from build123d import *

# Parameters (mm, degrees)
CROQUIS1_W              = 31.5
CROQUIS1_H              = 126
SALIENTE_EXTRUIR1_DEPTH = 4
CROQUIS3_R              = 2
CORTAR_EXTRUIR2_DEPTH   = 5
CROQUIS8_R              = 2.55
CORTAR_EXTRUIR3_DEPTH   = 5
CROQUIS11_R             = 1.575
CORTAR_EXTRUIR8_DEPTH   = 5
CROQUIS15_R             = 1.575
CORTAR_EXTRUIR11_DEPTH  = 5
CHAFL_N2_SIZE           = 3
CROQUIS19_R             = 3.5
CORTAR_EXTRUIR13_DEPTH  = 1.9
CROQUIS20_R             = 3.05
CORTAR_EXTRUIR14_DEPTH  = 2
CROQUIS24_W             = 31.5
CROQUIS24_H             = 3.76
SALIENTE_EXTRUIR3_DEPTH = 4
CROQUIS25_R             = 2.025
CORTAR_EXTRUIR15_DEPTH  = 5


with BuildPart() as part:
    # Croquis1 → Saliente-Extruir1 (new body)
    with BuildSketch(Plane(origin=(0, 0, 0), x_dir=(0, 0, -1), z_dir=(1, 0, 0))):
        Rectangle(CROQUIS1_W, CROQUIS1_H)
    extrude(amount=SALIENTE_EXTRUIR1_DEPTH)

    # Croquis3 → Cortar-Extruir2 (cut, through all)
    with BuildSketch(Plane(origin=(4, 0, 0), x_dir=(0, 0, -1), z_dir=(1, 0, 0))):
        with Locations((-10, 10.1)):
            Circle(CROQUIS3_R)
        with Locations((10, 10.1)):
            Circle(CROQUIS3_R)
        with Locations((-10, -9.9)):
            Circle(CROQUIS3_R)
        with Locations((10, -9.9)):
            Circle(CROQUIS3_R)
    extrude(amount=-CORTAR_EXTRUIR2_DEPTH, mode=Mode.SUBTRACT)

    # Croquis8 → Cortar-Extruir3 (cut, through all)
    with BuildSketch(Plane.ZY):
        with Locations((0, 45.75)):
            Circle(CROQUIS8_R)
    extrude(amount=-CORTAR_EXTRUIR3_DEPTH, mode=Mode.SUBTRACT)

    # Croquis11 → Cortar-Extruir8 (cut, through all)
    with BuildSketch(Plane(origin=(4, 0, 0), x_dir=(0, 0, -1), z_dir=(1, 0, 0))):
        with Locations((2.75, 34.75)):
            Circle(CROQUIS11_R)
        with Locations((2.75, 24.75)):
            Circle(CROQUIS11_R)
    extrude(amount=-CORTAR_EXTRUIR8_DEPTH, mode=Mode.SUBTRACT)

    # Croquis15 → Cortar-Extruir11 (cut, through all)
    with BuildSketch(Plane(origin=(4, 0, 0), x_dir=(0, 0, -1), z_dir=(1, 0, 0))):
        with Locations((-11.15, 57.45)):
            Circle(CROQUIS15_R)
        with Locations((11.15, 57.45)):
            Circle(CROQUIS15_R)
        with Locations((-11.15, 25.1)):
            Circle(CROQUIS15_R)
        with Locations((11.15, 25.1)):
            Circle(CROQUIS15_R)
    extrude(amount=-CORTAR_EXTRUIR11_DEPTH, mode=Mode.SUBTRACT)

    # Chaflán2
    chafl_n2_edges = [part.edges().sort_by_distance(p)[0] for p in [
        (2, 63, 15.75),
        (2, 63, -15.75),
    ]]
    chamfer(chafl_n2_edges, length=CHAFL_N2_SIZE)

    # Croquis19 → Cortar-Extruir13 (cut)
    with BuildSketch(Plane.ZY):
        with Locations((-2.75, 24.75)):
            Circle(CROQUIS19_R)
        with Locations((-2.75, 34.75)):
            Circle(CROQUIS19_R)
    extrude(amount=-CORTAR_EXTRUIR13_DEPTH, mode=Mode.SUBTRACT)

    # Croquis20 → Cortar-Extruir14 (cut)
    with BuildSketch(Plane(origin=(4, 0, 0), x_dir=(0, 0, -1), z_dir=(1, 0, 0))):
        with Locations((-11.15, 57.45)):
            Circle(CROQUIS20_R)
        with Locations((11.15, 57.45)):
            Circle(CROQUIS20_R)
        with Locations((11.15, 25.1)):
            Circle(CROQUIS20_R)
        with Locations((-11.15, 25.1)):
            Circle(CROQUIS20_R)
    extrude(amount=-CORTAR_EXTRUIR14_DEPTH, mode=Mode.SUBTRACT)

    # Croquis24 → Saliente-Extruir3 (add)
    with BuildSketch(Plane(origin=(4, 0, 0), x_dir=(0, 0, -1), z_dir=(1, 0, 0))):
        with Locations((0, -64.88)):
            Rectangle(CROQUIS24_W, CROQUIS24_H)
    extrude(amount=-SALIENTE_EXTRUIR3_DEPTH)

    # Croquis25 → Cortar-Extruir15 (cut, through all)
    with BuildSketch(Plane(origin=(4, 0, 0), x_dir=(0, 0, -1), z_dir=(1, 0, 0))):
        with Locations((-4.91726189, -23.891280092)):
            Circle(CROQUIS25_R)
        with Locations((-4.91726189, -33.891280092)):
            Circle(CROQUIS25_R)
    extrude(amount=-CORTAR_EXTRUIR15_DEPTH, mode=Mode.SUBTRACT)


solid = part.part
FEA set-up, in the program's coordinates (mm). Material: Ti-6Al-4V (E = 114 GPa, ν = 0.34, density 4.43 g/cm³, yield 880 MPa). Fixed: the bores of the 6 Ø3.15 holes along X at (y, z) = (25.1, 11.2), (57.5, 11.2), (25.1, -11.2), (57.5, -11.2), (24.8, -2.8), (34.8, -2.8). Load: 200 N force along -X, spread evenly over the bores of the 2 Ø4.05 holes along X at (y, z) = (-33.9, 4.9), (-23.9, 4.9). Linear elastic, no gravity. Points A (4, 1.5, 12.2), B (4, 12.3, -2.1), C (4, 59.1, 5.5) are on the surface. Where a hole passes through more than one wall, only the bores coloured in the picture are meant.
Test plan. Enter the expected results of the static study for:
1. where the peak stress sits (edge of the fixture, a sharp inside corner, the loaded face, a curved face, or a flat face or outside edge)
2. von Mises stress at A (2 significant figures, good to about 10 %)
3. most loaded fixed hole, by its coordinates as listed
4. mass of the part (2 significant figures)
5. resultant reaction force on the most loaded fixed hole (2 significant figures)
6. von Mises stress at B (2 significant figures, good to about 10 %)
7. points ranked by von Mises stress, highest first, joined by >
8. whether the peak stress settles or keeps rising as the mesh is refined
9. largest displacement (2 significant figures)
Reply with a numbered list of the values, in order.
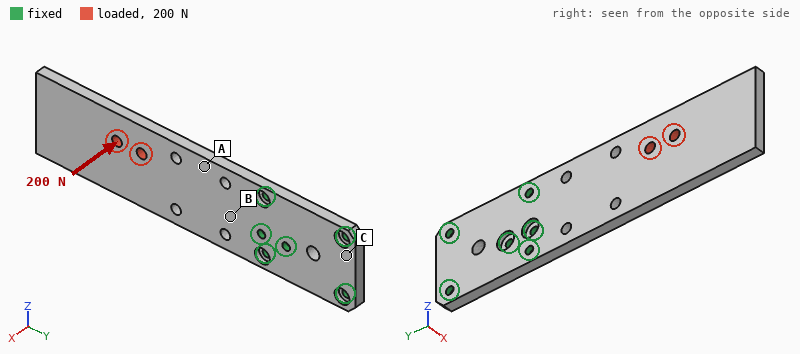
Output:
1. edge of the fixture
2. 71 MPa
3. (24.8, -2.8)
4. 68 g
5. 1.4 kN
6. 110 MPa
7. B > A > C
8. keeps rising
9. 1.4 mm
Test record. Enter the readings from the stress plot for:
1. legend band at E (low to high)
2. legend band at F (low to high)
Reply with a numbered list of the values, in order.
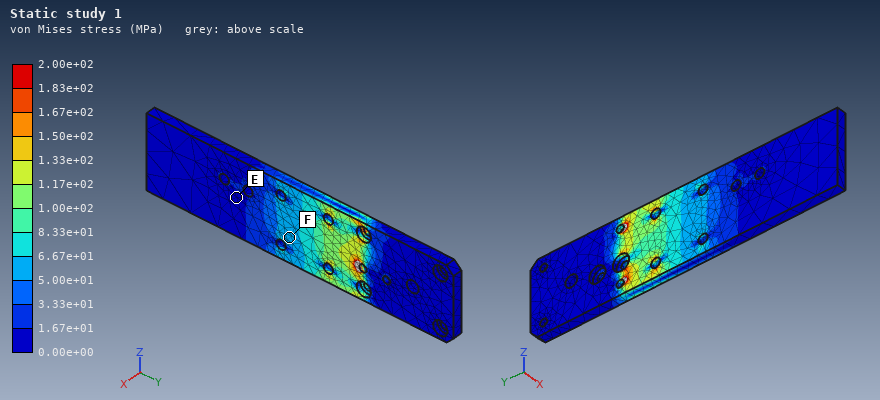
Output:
1. 0.00e+00 to 1.67e+01 MPa
2. 5.00e+01 to 6.67e+01 MPa
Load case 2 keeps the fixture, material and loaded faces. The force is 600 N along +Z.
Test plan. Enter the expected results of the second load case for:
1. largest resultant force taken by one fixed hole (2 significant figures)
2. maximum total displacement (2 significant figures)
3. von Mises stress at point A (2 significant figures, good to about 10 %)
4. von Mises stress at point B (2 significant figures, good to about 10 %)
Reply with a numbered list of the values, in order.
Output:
1. 1.2 kN
2. 85 µm
3. 20 MPa
4. 8.8 MPa
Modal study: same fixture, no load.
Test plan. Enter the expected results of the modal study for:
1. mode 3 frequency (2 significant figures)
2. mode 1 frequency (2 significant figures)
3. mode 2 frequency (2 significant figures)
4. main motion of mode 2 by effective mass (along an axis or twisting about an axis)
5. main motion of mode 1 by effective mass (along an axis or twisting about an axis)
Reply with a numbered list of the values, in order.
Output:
1. 2300 Hz
2. 360 Hz
3. 2100 Hz
4. twisting about Y
5. along X
